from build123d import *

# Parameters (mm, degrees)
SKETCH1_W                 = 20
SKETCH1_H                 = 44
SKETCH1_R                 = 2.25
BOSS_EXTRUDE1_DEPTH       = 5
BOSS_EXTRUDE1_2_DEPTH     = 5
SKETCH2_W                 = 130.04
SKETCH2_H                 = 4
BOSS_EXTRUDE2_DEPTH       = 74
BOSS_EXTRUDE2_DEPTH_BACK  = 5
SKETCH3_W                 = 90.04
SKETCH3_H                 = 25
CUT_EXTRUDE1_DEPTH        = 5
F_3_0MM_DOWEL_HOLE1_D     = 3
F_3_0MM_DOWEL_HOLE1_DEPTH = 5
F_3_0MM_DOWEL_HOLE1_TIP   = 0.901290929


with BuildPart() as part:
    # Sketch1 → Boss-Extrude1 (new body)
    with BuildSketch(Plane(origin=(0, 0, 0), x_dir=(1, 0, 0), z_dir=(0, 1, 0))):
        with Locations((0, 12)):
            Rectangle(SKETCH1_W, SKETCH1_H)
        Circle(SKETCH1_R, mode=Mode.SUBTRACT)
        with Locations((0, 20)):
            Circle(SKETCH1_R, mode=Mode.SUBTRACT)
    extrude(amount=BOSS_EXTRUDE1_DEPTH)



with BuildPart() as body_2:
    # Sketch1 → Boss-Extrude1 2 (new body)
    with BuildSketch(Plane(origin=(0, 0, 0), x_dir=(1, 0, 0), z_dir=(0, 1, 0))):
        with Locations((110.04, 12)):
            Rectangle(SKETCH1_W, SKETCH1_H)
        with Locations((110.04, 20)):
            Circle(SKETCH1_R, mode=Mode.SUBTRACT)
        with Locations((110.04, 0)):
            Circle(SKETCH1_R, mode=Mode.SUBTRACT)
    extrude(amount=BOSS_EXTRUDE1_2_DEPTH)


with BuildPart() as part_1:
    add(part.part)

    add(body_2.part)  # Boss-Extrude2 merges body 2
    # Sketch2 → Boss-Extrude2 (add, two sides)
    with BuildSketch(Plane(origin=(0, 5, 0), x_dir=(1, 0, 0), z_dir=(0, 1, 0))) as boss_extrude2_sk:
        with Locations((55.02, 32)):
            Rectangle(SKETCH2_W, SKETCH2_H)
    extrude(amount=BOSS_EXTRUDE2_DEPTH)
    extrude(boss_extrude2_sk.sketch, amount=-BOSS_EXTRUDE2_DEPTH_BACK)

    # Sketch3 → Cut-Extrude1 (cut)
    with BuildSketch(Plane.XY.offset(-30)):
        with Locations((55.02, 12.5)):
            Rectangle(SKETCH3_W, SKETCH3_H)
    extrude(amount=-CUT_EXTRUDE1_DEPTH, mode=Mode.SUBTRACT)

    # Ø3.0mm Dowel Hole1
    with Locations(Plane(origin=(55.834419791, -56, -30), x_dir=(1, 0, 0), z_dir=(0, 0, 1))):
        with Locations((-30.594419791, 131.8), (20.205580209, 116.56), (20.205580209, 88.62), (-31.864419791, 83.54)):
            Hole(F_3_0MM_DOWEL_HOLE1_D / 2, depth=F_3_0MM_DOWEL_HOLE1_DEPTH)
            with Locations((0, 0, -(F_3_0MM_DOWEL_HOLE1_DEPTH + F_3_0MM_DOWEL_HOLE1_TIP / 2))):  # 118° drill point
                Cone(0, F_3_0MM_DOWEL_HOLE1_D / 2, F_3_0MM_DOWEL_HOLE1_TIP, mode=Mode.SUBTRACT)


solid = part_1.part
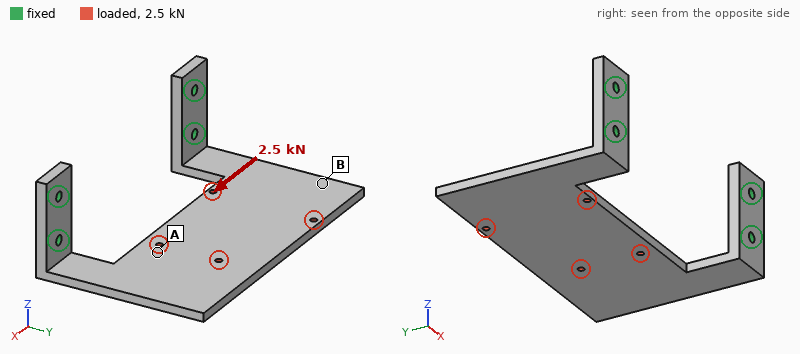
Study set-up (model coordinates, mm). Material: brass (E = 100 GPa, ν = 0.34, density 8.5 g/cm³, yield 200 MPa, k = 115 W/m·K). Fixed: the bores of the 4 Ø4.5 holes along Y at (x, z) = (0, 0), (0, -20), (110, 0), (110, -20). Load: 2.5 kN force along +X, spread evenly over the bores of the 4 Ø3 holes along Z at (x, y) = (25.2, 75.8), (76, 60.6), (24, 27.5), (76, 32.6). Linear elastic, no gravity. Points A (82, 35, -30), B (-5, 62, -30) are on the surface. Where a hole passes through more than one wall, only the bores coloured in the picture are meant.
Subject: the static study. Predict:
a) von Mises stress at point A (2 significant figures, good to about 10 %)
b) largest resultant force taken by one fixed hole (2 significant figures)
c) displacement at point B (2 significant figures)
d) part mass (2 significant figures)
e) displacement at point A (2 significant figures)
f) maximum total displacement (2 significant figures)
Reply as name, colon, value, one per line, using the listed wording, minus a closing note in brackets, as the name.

von Mises stress at point A: 24 MPa
largest resultant force taken by one fixed hole: 2.0 kN
displacement at point B: 0.13 mm
part mass: 340 g
displacement at point A: 0.091 mm
maximum total displacement: 0.15 mm
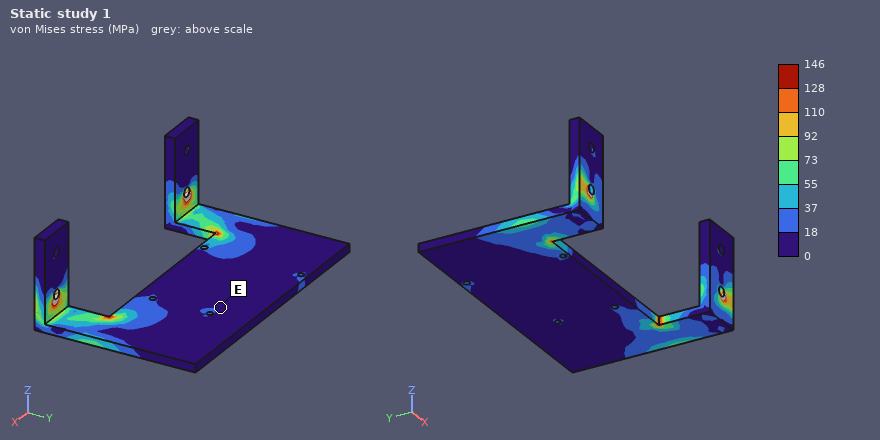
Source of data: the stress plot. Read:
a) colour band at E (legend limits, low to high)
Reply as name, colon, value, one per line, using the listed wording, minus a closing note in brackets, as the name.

colour band at E: 0 to 18 MPa
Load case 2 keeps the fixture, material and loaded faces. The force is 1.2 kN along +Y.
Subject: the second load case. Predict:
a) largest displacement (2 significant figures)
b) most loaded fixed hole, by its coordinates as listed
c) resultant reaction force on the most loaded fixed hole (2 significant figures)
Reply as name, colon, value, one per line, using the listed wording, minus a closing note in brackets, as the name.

largest displacement: 0.16 mm
most loaded fixed hole, by its coordinates as listed: (0, -20)
resultant reaction force on the most loaded fixed hole: 750 N
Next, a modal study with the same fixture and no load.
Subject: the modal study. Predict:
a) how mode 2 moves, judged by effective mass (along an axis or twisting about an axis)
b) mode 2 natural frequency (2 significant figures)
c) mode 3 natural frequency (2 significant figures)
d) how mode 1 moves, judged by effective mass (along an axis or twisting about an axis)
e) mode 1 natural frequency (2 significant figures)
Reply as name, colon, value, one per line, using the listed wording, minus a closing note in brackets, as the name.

how mode 2 moves, judged by effective mass: twisting about Y
mode 2 natural frequency: 530 Hz
mode 3 natural frequency: 980 Hz
how mode 1 moves, judged by effective mass: along Z
mode 1 natural frequency: 190 Hz
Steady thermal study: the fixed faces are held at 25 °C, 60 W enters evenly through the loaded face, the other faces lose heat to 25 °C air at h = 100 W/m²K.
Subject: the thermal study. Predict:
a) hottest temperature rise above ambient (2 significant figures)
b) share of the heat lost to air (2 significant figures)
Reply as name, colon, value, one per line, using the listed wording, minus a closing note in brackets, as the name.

hottest temperature rise above ambient: 54 K
share of the heat lost to air: 84 %
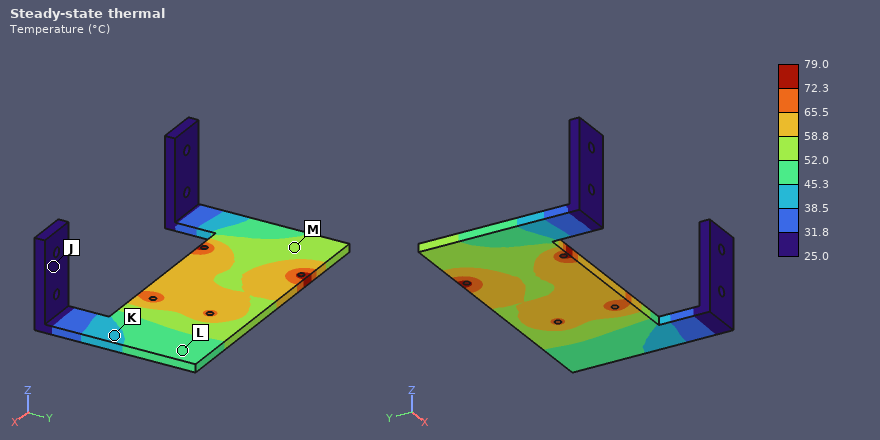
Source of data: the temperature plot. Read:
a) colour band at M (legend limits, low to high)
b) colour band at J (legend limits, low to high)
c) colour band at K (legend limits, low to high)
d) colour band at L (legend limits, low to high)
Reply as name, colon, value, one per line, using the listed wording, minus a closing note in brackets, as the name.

colour band at M: 52.0 to 58.8 °C
colour band at J: 25.0 to 31.8 °C
colour band at K: 38.5 to 45.3 °C
colour band at L: 45.3 to 52.0 °C
